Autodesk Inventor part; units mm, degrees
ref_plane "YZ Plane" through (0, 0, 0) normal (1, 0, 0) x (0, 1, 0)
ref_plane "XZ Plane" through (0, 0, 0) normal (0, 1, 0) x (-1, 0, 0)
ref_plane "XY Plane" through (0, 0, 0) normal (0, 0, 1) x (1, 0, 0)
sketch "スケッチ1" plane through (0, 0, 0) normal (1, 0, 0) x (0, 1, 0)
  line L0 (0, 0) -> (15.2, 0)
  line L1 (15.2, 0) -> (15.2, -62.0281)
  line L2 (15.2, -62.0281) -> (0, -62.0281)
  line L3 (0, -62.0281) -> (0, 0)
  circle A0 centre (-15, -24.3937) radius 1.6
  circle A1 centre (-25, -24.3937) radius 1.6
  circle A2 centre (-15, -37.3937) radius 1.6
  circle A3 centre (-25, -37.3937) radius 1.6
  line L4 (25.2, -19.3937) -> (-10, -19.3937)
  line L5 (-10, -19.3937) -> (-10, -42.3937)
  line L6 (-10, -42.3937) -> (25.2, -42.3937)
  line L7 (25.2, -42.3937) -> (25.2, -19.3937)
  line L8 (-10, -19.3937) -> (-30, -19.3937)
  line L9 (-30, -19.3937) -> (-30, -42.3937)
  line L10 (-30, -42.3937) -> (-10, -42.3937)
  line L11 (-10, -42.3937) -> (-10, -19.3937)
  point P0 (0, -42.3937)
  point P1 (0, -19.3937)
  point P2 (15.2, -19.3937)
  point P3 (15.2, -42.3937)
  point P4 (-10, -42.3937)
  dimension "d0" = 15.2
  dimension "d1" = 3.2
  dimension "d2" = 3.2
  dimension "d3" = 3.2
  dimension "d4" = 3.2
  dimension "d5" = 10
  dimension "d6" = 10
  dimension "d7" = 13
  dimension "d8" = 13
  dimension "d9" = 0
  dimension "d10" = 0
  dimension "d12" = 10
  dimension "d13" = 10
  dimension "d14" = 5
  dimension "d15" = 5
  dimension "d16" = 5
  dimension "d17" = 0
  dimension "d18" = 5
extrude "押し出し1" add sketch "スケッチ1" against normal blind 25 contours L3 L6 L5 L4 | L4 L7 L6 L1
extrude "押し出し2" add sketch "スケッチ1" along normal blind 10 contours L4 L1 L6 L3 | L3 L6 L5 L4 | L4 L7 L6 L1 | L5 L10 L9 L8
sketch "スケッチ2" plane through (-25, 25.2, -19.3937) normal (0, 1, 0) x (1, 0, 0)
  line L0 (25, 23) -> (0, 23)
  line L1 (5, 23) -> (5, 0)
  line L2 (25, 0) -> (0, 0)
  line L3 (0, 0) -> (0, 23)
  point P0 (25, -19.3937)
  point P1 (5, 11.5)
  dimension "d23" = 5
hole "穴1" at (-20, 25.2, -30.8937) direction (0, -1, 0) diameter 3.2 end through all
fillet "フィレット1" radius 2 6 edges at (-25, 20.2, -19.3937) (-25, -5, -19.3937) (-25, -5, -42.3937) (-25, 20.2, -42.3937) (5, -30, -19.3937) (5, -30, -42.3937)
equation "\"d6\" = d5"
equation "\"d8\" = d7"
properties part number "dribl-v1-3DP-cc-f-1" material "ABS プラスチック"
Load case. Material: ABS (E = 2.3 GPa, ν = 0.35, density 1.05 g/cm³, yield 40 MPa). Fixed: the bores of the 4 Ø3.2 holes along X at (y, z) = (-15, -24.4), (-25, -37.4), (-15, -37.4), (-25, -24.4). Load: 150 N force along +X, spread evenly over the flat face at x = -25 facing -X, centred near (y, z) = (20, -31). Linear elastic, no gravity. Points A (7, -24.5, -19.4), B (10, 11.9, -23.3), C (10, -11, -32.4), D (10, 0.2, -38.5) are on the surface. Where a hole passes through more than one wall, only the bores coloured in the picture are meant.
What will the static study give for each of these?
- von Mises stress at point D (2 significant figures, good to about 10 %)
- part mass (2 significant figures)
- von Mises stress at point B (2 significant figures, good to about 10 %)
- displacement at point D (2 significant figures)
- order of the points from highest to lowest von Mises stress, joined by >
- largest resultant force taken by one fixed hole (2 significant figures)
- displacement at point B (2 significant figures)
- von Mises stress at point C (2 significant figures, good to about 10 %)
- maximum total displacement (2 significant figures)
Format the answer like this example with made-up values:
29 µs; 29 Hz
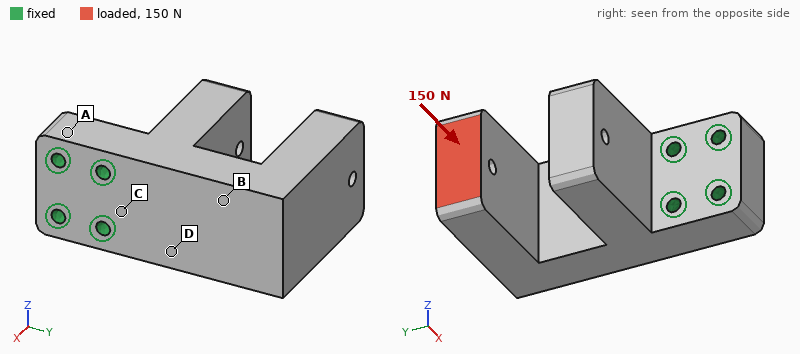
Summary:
6.7 MPa; 25 g; 3.2 MPa; 0.14 mm; C > D > B > A; 110 N; 0.32 mm; 8.4 MPa; 0.79 mm
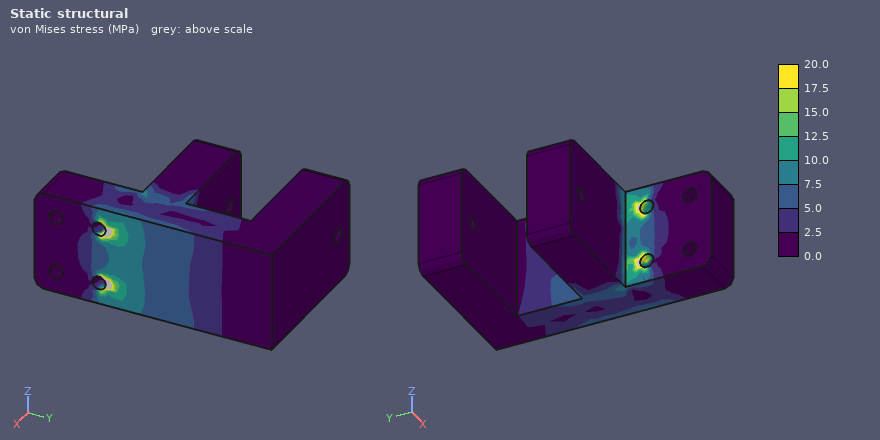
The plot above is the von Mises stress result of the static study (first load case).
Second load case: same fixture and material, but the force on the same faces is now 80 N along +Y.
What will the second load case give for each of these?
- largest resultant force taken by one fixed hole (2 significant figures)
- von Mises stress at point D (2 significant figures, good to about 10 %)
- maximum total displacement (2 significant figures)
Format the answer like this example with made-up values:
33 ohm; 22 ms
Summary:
40 N; 5.1 MPa; 0.75 mm
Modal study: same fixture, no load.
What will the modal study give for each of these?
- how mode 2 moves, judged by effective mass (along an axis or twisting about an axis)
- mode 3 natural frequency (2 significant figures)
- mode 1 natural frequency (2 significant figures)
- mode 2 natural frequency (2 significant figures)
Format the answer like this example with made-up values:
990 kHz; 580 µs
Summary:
along Z; 1900 Hz; 750 Hz; 1200 Hz
